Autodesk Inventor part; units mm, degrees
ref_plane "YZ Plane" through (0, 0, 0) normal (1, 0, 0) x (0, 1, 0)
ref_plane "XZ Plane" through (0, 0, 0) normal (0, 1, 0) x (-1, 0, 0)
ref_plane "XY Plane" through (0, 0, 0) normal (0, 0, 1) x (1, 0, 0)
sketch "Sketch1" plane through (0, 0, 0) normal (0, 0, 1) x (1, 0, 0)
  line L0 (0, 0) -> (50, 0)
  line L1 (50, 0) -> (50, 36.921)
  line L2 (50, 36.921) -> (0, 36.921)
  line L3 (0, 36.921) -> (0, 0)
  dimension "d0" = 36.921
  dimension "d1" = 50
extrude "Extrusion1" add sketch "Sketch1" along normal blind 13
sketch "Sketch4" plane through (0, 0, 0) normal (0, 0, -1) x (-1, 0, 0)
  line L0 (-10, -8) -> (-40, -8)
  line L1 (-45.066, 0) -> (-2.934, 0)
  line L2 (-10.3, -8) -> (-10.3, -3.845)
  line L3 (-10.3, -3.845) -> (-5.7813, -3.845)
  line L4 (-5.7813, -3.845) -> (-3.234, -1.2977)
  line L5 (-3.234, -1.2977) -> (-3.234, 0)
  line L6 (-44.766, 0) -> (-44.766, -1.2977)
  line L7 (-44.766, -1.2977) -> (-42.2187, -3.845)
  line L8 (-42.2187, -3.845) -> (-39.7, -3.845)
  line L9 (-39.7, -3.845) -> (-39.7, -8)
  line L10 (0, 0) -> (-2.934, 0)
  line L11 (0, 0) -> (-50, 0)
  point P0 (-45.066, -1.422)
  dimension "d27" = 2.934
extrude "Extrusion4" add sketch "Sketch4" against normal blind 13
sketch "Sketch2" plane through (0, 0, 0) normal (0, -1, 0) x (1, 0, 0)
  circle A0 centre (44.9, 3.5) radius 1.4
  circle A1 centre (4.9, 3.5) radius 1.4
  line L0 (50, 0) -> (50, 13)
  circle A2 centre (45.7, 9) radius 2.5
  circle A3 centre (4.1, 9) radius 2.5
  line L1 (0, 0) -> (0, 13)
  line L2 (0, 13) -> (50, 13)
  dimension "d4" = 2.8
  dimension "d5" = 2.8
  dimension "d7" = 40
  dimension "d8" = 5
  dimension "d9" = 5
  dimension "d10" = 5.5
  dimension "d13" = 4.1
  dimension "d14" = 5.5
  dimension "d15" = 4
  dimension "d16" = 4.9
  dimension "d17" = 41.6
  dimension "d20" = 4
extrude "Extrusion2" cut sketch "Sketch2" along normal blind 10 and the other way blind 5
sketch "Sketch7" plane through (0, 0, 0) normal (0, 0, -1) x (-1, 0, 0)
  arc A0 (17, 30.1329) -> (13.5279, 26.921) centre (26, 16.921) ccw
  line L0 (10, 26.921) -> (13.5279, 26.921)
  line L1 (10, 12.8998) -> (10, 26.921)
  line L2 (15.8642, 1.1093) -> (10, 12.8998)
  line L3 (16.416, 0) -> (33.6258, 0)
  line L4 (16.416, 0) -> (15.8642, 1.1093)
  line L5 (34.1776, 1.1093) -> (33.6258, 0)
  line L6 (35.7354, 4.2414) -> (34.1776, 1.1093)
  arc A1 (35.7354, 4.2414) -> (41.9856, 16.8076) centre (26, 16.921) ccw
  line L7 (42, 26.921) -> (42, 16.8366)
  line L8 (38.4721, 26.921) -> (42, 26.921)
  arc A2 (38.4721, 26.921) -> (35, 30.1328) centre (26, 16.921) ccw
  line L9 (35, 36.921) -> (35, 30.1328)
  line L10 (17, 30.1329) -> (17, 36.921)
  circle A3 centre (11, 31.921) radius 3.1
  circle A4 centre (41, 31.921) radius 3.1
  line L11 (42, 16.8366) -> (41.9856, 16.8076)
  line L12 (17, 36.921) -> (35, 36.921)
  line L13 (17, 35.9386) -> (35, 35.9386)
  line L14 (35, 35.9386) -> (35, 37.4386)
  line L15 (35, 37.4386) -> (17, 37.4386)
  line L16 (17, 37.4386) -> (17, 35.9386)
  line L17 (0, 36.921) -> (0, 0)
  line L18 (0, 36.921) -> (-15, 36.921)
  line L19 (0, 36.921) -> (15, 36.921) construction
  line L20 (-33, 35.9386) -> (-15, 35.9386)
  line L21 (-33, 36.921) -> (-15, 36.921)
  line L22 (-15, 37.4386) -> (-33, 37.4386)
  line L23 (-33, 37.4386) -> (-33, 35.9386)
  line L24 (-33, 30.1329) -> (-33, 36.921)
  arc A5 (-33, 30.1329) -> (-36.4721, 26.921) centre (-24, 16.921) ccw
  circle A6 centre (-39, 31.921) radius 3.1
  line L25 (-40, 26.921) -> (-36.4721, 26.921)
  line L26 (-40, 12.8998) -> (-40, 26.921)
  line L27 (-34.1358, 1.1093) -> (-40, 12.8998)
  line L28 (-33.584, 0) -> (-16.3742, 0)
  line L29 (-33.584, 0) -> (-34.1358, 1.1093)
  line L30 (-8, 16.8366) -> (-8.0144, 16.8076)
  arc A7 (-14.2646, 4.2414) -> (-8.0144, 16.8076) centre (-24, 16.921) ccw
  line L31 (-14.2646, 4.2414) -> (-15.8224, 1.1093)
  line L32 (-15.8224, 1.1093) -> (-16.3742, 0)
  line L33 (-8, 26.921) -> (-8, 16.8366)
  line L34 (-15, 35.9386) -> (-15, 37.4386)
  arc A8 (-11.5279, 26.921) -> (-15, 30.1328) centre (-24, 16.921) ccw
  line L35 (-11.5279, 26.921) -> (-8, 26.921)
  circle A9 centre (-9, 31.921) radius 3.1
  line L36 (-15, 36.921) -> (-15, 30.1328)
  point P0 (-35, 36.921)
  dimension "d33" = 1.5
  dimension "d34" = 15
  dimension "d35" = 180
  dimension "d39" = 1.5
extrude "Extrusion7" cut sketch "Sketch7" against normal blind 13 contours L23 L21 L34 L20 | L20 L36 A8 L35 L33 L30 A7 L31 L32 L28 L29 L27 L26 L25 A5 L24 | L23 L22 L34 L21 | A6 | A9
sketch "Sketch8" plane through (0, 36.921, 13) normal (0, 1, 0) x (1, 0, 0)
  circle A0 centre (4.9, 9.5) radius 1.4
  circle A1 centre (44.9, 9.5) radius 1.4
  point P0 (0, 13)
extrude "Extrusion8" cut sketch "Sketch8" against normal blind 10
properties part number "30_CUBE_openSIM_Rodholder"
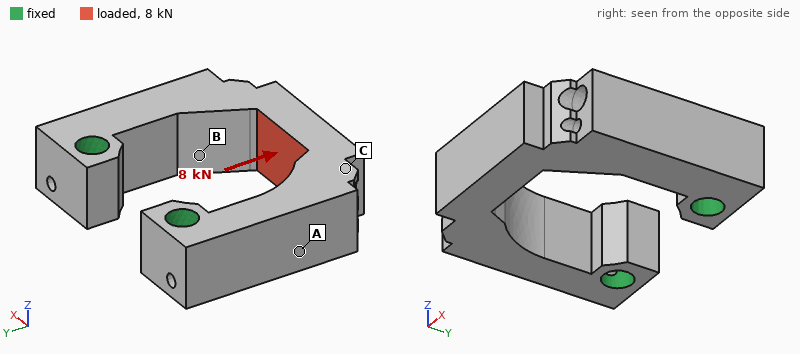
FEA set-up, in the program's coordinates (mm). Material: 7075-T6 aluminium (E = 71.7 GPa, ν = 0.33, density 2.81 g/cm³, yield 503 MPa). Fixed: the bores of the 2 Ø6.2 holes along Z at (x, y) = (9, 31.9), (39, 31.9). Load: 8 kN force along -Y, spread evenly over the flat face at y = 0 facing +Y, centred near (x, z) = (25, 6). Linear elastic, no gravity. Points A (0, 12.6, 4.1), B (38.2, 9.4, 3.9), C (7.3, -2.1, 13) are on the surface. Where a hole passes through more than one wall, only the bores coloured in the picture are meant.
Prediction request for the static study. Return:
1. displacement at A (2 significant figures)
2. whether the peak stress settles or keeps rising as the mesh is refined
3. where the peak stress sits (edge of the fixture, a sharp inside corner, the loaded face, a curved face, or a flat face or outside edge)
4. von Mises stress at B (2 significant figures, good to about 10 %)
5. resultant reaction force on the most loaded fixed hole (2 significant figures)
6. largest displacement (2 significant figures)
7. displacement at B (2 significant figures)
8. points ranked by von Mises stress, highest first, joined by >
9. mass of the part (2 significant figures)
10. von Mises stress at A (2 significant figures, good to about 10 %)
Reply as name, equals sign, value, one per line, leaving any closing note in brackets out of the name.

displacement at A = 37 µm
whether the peak stress settles or keeps rising as the mesh is refined = keeps rising
where the peak stress sits = edge of the fixture
von Mises stress at B = 120 MPa
resultant reaction force on the most loaded fixed hole = 4.4 kN
largest displacement = 85 µm
displacement at B = 39 µm
points ranked by von Mises stress, highest first, joined by > = B > A > C
mass of the part = 39 g
von Mises stress at A = 62 MPa
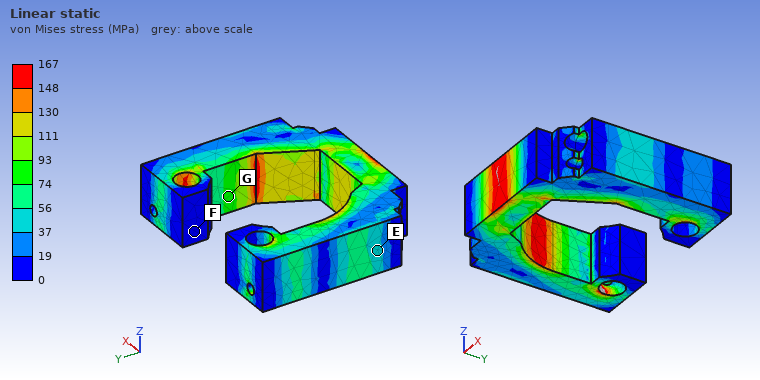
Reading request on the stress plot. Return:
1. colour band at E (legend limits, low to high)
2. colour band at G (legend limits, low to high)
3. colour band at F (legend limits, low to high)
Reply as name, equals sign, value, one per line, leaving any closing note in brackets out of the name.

colour band at E = 37 to 56 MPa
colour band at G = 74 to 93 MPa
colour band at F = 0 to 19 MPa
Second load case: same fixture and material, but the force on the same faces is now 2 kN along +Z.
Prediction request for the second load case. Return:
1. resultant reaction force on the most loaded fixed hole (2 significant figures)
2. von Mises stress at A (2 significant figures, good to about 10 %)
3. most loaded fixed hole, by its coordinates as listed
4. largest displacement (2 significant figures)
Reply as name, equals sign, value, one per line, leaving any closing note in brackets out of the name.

resultant reaction force on the most loaded fixed hole = 1.1 kN
von Mises stress at A = 16 MPa
most loaded fixed hole, by its coordinates as listed = (39, 31.9)
largest displacement = 0.17 mm
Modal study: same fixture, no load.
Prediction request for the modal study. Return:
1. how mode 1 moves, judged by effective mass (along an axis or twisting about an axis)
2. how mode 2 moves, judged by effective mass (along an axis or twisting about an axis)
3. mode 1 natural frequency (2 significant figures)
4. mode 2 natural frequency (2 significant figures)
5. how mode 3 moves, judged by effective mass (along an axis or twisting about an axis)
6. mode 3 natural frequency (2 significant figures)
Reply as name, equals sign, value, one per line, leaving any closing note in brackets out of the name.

how mode 1 moves, judged by effective mass = along Z
how mode 2 moves, judged by effective mass = along X
mode 1 natural frequency = 4600 Hz
mode 2 natural frequency = 5800 Hz
how mode 3 moves, judged by effective mass = twisting about Y
mode 3 natural frequency = 9600 Hz
